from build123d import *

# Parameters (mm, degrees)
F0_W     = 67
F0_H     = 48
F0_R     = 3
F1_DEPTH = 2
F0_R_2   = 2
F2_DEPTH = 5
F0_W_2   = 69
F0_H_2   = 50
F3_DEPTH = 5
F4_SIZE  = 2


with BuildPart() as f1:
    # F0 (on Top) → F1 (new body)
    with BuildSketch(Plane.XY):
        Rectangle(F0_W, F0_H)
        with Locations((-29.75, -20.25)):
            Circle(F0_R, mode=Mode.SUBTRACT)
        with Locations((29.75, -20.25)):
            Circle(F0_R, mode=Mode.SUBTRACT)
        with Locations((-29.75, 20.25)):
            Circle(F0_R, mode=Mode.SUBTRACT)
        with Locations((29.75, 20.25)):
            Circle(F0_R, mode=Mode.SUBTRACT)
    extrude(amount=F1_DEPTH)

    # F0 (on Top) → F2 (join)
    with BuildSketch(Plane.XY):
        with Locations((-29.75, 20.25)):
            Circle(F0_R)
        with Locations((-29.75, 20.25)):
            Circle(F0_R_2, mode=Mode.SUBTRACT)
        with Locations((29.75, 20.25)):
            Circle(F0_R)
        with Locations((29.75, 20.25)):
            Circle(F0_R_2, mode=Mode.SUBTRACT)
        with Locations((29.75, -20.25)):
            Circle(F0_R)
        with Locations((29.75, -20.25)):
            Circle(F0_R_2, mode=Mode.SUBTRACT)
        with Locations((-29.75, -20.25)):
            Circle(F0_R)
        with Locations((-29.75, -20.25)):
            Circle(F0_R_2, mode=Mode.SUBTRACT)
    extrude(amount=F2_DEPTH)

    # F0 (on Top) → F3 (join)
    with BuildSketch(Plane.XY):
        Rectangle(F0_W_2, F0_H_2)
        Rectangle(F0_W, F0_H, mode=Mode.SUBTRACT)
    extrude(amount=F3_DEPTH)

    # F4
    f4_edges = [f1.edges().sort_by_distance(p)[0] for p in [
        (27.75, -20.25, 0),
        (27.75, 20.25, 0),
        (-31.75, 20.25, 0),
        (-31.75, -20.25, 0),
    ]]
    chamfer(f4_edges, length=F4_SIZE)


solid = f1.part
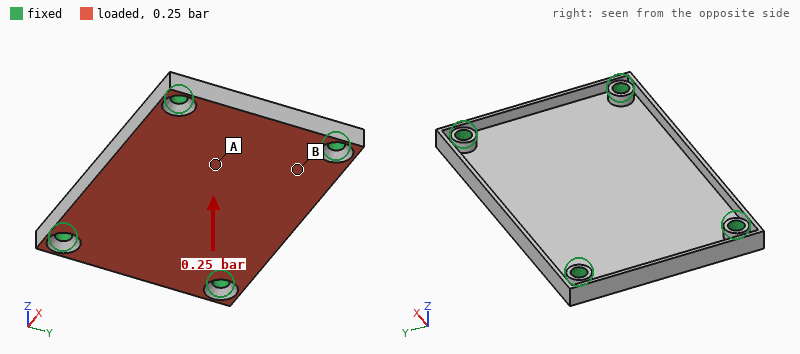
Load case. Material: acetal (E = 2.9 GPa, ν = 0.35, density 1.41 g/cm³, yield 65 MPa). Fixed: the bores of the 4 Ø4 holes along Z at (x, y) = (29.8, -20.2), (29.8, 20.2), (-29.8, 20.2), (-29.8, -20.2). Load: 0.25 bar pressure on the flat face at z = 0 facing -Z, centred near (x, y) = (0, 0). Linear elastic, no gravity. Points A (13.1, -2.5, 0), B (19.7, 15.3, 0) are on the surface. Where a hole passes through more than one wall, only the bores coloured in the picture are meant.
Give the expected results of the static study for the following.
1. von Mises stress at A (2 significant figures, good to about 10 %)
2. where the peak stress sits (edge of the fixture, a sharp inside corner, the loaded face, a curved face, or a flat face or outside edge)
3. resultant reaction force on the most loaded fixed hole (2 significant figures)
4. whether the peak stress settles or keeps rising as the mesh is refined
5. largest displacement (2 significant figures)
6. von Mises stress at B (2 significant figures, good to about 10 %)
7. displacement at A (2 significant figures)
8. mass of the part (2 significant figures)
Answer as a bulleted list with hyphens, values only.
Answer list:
- 4.2 MPa
- a sharp inside corner
- 43 N
- keeps rising
- 0.49 mm
- 1.7 MPa
- 0.38 mm
- 11 g
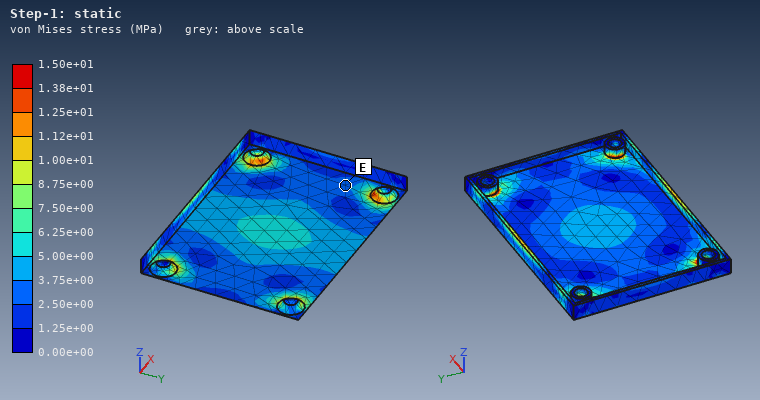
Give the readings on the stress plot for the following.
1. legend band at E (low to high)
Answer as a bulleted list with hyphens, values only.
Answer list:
- 2.50e+00 to 3.75e+00 MPa
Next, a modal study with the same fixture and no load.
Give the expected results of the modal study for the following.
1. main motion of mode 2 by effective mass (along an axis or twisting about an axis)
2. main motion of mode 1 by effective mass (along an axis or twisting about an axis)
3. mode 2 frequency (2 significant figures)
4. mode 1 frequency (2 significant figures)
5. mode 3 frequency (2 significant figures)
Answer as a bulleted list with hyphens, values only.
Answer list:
- twisting about X
- along Z
- 1200 Hz
- 810 Hz
- 1800 Hz
